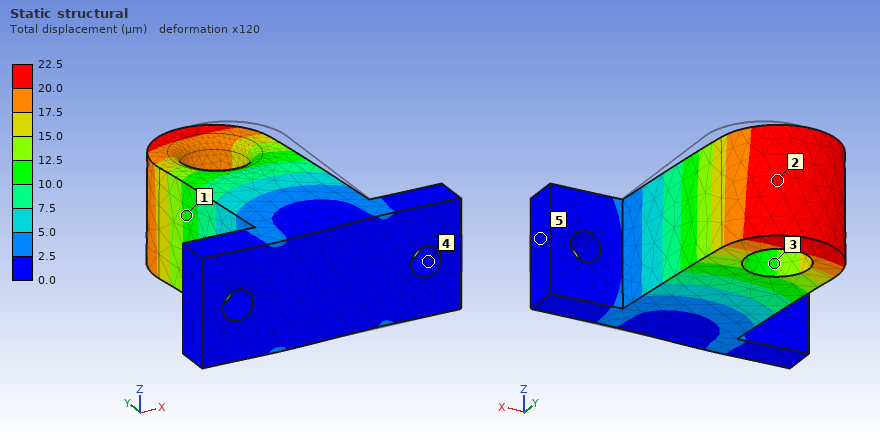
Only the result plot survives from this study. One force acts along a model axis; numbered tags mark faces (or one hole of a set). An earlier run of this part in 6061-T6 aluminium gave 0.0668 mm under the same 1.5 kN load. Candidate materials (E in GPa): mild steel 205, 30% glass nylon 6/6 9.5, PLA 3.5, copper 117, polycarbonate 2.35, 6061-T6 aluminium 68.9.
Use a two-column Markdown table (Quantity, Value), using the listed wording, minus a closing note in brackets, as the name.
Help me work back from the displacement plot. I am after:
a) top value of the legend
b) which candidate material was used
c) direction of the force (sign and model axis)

| Quantity | Value |
|---|---|
| top value of the legend | 22.5 µm |
| which candidate material was used | mild steel |
| direction of the force | -X |
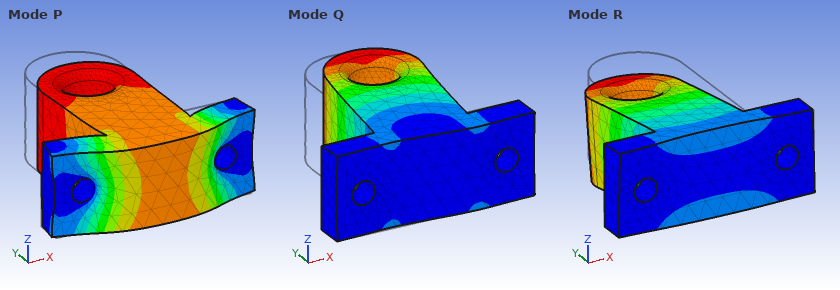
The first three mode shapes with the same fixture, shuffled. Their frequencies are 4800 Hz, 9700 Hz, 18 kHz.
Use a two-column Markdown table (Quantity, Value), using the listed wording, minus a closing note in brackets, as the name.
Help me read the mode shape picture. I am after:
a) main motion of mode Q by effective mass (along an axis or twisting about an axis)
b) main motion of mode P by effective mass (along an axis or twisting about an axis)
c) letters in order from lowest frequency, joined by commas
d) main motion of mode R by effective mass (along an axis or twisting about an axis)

| Quantity | Value |
|---|---|
| main motion of mode Q by effective mass | along X |
| main motion of mode P by effective mass | along Y |
| letters in order from lowest frequency, joined by commas | R, Q, P |
| main motion of mode R by effective mass | along Z |
